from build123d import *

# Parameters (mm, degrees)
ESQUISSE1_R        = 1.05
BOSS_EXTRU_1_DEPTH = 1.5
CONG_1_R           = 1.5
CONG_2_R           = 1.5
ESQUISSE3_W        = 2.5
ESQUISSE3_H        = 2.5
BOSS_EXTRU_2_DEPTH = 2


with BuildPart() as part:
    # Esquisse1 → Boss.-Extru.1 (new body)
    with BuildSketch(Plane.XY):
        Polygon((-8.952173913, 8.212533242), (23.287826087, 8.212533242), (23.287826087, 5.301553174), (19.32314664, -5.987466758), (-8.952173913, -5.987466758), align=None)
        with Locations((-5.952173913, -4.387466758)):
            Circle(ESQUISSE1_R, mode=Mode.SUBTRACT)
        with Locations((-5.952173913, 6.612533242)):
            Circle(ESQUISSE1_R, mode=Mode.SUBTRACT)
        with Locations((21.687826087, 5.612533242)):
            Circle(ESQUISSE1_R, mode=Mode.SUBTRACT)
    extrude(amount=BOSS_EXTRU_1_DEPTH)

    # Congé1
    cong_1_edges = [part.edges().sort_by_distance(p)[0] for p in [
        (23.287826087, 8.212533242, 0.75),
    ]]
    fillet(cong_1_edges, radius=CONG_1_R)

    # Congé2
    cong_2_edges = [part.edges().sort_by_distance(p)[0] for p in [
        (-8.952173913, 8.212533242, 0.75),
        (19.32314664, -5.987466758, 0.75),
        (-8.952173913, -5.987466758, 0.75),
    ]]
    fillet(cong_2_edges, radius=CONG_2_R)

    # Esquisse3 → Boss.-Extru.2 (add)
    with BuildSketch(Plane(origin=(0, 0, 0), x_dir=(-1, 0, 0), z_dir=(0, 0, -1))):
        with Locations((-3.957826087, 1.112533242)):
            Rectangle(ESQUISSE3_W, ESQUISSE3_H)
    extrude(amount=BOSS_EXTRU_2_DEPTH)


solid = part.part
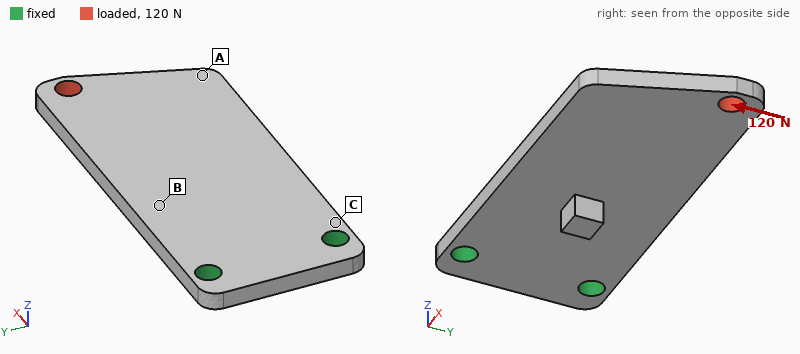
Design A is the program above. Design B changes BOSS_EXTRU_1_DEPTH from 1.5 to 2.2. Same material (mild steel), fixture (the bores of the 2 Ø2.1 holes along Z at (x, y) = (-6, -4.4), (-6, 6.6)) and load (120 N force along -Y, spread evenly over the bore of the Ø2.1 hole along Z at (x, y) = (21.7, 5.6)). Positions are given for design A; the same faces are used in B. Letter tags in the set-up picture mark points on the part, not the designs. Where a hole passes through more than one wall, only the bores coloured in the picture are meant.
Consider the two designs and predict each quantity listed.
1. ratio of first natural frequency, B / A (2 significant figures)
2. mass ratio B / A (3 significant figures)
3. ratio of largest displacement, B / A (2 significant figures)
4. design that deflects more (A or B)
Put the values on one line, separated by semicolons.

1.4; 1.46; 0.68; A
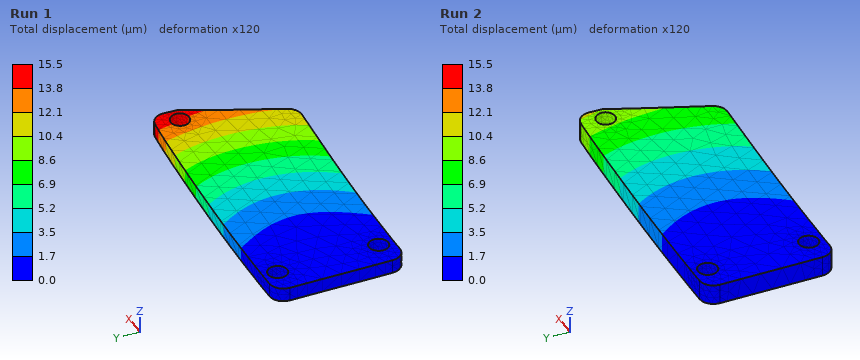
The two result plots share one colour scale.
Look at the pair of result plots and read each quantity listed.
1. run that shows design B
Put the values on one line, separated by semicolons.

Run 2
